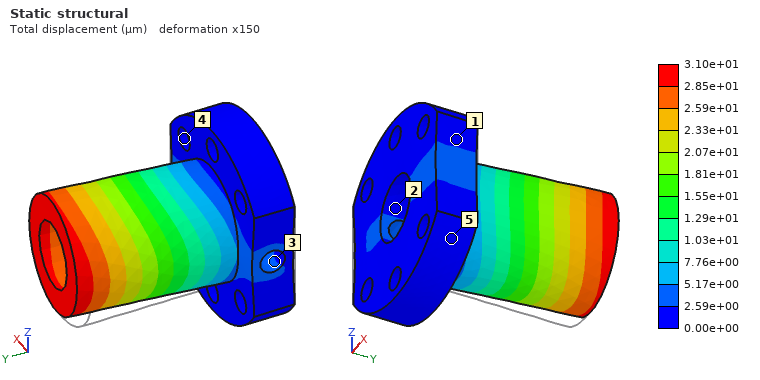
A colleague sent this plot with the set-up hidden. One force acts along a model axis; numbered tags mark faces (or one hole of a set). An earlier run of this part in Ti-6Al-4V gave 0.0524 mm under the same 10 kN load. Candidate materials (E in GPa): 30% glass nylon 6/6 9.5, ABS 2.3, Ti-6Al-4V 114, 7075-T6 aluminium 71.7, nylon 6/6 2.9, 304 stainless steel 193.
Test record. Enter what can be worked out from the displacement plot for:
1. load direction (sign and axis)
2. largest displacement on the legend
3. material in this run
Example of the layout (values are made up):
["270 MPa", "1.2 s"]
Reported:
["+X", "3.10e+01 µm", "304 stainless steel"]
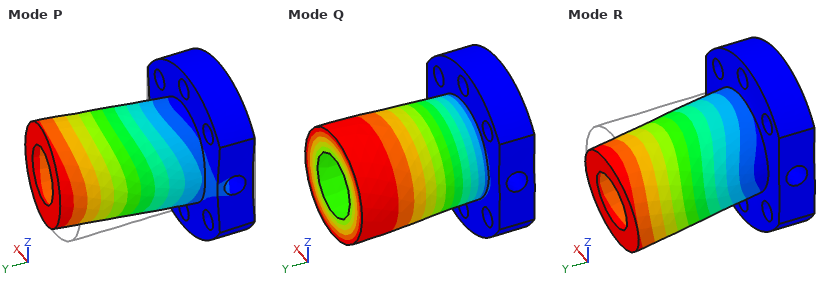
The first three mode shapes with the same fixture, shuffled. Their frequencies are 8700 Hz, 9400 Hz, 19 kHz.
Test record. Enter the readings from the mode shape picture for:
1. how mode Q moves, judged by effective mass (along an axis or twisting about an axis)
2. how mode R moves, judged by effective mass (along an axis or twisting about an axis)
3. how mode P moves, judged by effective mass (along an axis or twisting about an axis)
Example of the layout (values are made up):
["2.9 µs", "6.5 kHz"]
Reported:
["twisting about Y", "along Z", "along X"]
